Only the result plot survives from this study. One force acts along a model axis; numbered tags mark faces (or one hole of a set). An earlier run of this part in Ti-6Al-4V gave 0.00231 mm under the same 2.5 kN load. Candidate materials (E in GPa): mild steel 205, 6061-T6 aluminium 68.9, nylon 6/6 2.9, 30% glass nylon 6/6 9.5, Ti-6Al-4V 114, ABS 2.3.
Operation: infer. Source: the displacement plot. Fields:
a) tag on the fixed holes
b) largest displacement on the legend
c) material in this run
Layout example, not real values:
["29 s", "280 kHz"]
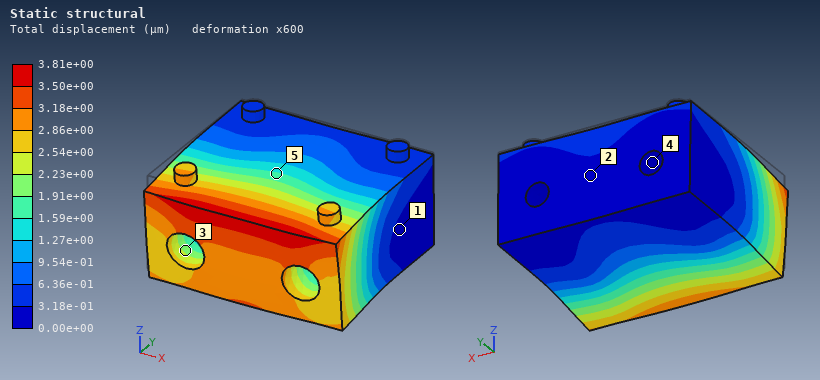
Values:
["4", "3.81e+00 µm", "6061-T6 aluminium"]
